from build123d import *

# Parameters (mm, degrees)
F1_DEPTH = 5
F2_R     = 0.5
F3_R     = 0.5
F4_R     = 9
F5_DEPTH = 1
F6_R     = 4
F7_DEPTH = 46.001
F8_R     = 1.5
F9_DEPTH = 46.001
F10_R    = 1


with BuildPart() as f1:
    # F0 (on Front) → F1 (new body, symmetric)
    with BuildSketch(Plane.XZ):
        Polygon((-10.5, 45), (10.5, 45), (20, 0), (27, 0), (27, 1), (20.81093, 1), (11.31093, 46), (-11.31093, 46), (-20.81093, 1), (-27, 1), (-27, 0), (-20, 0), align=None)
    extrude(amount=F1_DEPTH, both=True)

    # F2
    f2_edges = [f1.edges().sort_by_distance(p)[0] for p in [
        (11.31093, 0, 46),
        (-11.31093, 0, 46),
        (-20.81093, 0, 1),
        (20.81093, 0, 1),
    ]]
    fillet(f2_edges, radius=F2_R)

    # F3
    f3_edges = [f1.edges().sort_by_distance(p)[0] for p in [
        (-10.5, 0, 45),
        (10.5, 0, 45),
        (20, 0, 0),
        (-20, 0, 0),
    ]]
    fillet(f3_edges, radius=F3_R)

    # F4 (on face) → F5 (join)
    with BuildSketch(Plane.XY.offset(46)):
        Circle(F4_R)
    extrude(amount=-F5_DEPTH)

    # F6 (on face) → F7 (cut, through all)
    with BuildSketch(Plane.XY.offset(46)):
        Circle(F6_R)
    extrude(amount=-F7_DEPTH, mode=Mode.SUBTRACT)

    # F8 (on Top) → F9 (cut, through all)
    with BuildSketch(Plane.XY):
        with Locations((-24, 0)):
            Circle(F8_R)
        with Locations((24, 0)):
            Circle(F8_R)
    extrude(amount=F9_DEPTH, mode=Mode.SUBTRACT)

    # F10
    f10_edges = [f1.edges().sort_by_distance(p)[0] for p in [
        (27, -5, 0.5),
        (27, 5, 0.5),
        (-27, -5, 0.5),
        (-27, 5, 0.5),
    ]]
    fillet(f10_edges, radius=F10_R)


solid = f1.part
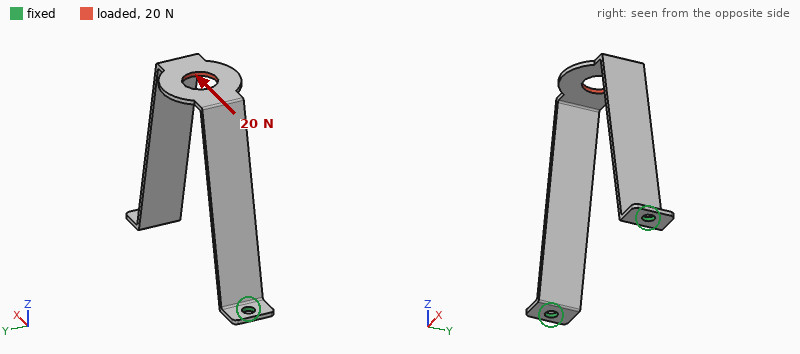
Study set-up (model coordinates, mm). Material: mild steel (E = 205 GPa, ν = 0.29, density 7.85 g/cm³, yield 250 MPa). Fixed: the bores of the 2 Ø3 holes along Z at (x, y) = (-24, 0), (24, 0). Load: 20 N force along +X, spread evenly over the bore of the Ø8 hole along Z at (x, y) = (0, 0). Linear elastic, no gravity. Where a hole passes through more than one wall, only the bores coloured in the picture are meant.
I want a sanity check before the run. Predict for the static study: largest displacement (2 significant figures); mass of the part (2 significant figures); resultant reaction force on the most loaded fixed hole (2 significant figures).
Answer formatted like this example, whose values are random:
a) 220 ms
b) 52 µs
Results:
a) 0.29 mm
b) 10 g
c) 18 N
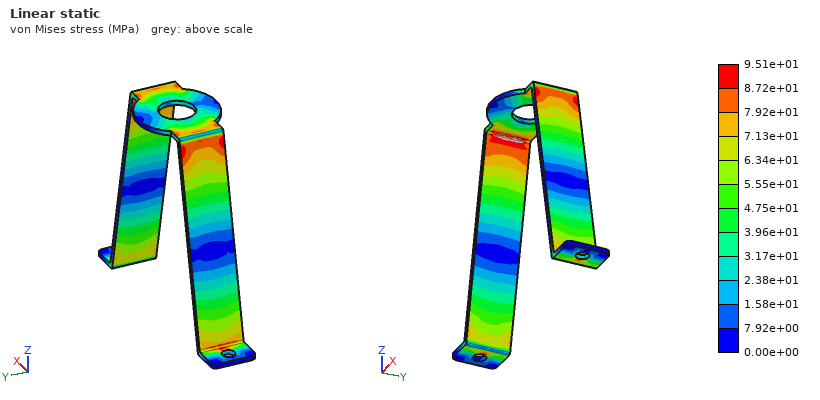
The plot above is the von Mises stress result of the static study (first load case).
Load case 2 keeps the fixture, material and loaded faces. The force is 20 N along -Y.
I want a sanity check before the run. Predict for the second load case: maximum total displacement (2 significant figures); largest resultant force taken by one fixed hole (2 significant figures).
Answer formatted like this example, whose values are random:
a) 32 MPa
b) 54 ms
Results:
a) 0.15 mm
b) 10 N
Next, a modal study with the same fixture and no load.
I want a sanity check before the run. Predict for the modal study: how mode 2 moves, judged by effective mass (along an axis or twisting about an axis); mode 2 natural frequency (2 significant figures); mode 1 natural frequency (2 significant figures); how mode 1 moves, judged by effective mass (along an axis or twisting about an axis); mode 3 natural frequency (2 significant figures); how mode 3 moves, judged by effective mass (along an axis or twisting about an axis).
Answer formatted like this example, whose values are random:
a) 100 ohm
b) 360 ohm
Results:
a) along Y
b) 900 Hz
c) 580 Hz
d) along X
e) 1500 Hz
f) twisting about Z
